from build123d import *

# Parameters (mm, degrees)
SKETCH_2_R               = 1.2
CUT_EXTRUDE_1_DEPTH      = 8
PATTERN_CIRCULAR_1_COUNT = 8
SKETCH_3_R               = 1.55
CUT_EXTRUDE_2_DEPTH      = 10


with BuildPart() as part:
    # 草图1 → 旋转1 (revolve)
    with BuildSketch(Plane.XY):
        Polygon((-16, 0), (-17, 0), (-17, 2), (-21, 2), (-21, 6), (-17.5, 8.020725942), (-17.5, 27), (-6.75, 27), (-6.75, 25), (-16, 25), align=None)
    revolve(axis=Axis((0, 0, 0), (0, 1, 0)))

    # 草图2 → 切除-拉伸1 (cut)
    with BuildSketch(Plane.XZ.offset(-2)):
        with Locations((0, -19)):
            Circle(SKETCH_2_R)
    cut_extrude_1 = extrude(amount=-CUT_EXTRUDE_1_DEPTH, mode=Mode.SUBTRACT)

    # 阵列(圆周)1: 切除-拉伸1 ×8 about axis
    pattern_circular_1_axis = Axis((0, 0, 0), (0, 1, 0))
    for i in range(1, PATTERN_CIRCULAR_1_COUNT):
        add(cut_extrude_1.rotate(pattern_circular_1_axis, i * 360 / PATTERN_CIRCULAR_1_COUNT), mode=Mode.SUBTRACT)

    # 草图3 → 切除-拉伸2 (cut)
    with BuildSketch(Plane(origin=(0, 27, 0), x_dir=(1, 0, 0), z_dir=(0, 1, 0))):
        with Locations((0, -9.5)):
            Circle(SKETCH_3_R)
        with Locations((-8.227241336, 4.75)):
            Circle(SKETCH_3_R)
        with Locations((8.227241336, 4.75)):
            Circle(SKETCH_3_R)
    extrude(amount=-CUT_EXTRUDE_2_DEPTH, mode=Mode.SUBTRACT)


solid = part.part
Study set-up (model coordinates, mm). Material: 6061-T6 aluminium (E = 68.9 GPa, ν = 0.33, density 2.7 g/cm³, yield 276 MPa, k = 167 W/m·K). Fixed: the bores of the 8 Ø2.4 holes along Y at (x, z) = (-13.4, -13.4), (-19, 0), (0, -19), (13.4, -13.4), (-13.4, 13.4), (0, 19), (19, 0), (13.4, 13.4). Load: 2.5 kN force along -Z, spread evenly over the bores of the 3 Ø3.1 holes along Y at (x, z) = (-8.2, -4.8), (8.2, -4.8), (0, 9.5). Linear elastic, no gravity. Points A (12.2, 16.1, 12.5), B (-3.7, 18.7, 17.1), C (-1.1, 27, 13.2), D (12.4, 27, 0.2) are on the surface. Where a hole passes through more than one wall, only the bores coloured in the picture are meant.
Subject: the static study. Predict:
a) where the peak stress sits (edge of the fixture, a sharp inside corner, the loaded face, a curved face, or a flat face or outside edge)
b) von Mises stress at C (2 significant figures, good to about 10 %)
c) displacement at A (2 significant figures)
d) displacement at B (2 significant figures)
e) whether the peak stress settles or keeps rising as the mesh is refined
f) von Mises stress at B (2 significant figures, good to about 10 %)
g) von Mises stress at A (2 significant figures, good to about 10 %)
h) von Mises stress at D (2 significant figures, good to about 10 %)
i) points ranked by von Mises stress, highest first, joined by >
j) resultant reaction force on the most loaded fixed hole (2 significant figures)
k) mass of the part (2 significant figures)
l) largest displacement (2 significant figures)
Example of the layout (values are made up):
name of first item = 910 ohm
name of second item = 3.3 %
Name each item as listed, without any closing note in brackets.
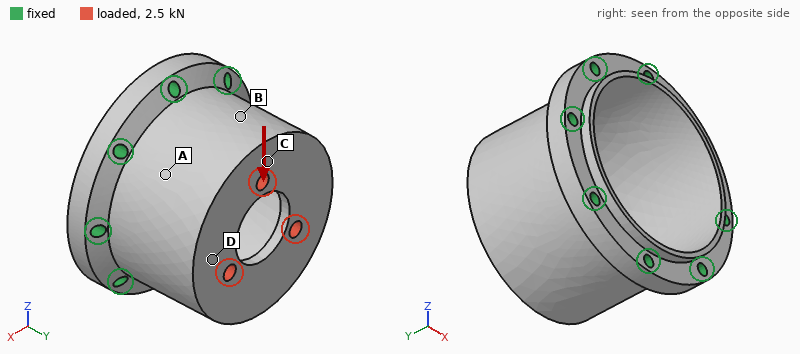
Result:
where the peak stress sits = edge of the fixture
von Mises stress at C = 58 MPa
displacement at A = 14 µm
displacement at B = 20 µm
whether the peak stress settles or keeps rising as the mesh is refined = keeps rising
von Mises stress at B = 25 MPa
von Mises stress at A = 39 MPa
von Mises stress at D = 18 MPa
points ranked by von Mises stress, highest first, joined by > = C > A > B > D
resultant reaction force on the most loaded fixed hole = 740 N
mass of the part = 20 g
largest displacement = 49 µm
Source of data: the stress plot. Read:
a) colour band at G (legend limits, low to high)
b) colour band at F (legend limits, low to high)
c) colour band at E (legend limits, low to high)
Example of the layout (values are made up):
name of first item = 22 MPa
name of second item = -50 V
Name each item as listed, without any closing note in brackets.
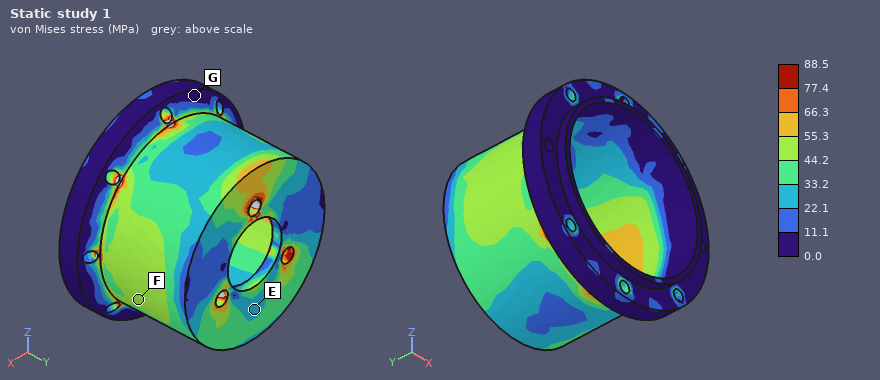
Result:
colour band at G = 0.0 to 11.1 MPa
colour band at F = 44.2 to 55.3 MPa
colour band at E = 22.1 to 33.2 MPa
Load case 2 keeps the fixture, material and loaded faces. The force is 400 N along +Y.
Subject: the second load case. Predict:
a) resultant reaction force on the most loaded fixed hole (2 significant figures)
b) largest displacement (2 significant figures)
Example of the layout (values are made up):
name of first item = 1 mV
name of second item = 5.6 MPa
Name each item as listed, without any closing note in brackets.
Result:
resultant reaction force on the most loaded fixed hole = 55 N
largest displacement = 36 µm
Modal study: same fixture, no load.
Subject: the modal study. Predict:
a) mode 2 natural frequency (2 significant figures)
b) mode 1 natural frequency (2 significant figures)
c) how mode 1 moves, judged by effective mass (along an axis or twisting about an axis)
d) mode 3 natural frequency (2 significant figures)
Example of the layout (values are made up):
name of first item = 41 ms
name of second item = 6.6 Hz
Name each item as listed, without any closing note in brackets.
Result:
mode 2 natural frequency = 17 kHz
mode 1 natural frequency = 16 kHz
how mode 1 moves, judged by effective mass = along Y
mode 3 natural frequency = 17 kHz
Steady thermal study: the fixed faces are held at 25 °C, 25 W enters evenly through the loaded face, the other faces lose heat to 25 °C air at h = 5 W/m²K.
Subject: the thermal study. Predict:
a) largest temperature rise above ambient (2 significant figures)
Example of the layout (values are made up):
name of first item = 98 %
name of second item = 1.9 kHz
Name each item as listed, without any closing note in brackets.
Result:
largest temperature rise above ambient = 31 K
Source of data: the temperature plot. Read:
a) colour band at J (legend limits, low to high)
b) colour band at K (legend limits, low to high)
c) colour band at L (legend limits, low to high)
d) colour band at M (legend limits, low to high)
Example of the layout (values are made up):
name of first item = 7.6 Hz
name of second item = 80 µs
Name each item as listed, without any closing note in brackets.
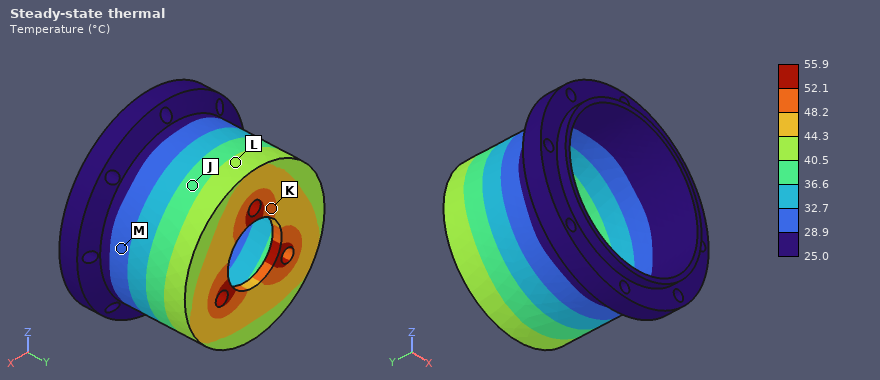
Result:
colour band at J = 36.6 to 40.5 °C
colour band at K = 48.2 to 52.1 °C
colour band at L = 40.5 to 44.3 °C
colour band at M = 28.9 to 32.7 °C
